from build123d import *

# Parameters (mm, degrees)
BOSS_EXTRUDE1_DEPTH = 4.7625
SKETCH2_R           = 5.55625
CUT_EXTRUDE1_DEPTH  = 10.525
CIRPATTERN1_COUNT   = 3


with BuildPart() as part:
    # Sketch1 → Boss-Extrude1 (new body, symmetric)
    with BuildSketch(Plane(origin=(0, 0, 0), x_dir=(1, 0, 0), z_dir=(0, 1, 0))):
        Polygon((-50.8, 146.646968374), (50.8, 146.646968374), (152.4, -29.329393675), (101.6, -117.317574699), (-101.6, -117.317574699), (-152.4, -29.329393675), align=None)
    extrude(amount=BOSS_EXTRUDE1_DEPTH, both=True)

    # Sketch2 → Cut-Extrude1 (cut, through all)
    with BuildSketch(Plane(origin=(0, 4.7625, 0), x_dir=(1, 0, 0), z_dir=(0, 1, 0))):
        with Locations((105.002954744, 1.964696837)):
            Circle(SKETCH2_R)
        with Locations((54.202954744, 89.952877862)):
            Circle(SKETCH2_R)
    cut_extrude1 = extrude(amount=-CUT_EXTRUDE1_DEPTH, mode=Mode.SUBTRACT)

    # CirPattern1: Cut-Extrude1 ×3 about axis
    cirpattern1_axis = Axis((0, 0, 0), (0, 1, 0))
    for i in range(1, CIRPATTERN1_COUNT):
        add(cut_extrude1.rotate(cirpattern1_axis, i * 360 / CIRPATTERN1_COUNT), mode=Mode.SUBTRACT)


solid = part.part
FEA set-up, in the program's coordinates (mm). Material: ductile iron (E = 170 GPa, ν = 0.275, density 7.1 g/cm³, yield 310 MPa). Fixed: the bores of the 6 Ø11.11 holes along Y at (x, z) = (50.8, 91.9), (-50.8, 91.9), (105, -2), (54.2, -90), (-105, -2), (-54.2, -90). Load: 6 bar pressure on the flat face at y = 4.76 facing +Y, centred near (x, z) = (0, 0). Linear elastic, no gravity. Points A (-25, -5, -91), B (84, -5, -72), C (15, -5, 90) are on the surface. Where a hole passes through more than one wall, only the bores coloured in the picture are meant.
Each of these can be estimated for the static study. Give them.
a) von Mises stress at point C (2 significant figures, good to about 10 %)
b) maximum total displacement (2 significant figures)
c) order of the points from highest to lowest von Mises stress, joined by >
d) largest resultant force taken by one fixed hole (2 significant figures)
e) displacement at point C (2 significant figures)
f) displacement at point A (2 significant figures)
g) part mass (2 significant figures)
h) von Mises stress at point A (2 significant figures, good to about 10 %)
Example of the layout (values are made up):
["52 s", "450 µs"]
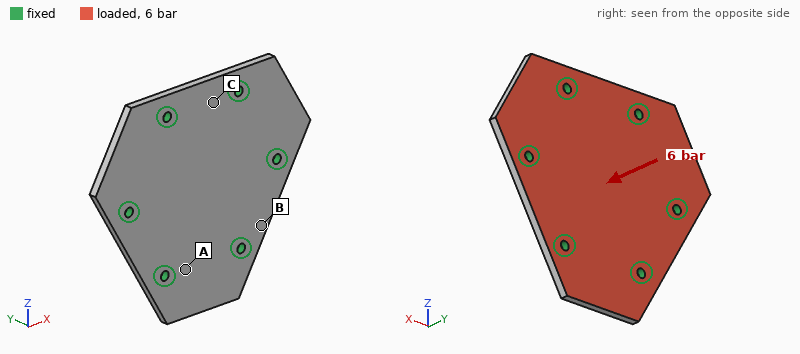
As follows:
["24 MPa", "0.10 mm", "A > C > B", "5.8 kN", "0.018 mm", "0.023 mm", "3.9 kg", "41 MPa"]
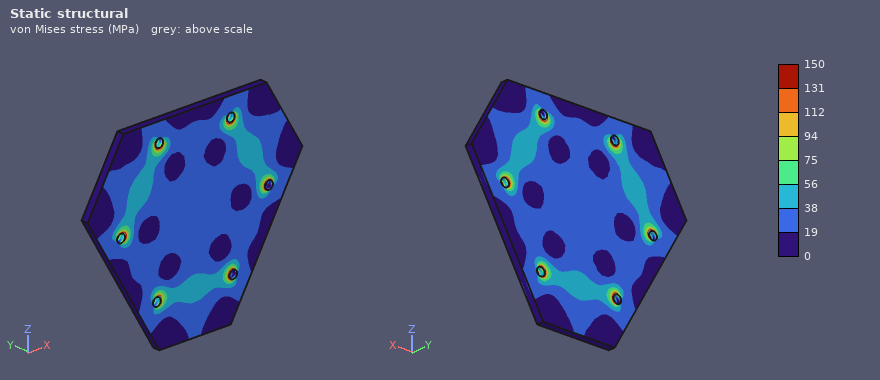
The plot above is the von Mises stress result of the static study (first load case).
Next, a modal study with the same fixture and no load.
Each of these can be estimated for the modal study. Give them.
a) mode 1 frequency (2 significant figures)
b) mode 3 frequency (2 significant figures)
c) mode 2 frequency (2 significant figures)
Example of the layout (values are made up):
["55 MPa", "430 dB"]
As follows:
["1700 Hz", "2000 Hz", "2000 Hz"]
